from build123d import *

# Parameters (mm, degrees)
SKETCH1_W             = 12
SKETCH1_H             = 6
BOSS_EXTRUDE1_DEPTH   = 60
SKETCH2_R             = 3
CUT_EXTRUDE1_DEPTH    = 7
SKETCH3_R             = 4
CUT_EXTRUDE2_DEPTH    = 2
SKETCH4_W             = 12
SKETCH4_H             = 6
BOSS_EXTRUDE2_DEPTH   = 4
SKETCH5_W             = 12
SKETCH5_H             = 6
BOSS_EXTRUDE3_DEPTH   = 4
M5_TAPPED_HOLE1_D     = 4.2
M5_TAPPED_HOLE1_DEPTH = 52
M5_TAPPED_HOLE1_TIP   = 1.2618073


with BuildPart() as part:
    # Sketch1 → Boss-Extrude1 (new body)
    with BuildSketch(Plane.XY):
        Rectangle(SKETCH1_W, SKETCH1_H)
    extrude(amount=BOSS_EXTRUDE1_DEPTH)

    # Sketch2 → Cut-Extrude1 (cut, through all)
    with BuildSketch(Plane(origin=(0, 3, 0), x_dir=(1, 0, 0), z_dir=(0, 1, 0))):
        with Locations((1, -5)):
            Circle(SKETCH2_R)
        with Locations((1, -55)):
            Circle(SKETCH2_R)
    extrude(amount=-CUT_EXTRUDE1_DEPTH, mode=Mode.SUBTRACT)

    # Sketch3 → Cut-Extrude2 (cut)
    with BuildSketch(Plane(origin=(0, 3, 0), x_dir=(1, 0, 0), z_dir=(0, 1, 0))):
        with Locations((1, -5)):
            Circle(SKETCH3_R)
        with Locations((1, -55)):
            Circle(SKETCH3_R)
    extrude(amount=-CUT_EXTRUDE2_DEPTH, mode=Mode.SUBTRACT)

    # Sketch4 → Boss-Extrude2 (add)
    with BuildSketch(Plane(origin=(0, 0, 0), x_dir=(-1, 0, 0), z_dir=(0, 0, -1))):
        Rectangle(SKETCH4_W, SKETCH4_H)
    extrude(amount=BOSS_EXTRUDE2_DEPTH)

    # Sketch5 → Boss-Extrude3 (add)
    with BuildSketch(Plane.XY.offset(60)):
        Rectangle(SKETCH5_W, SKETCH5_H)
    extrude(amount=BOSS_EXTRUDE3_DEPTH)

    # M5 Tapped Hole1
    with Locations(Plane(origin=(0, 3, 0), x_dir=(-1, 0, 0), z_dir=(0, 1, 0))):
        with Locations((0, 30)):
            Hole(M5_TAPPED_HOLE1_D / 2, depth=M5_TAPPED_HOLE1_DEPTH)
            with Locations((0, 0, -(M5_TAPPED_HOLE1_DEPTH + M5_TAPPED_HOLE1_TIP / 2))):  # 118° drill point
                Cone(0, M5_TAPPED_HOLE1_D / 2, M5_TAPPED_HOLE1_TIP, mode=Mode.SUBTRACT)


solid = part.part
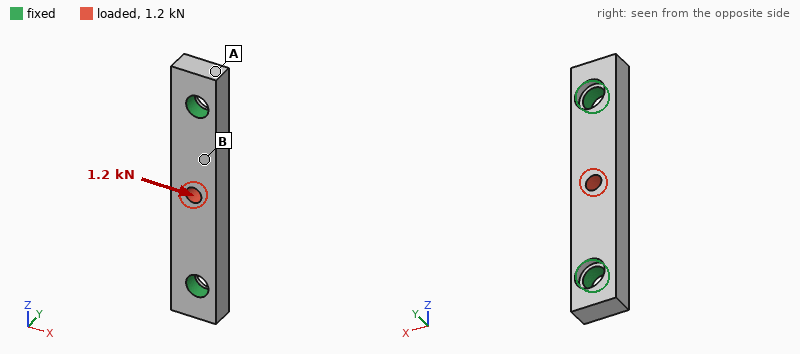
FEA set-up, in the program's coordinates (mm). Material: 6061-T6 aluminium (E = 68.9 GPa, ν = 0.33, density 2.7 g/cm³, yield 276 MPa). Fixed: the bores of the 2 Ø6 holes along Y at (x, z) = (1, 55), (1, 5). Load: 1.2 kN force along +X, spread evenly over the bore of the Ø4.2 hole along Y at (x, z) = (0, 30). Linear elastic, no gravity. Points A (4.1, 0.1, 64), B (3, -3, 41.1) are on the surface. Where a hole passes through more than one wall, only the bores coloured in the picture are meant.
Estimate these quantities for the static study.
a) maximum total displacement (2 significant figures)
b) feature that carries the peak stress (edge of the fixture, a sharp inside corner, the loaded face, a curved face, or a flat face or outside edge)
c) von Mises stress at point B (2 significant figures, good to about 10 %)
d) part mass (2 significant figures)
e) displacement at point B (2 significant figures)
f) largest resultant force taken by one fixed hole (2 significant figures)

25 µm
edge of the fixture
17 MPa
12 g
15 µm
610 N
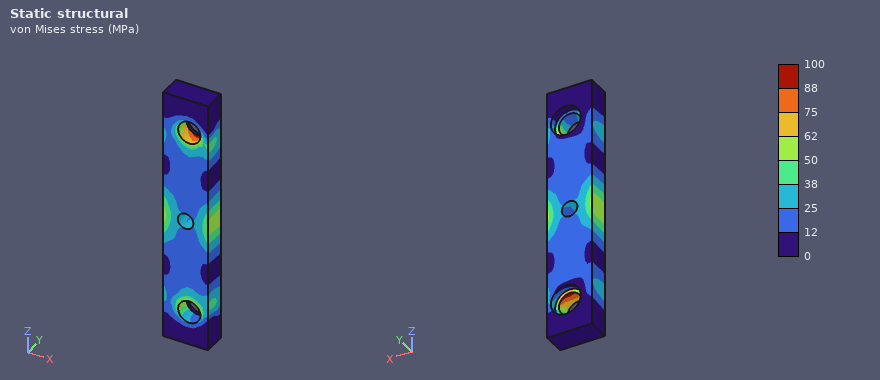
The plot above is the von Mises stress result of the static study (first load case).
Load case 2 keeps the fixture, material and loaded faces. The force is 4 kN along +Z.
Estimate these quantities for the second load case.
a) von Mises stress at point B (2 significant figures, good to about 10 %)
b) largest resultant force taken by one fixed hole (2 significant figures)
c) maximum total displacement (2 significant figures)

36 MPa
2.0 kN
12 µm
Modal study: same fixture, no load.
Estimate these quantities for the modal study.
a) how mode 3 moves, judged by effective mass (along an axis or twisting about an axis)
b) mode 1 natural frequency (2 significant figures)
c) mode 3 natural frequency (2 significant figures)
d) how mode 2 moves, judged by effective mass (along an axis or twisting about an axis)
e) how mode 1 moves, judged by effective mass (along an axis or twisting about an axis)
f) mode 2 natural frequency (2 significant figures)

twisting about Z
11 kHz
23 kHz
along X
along Y
18 kHz
